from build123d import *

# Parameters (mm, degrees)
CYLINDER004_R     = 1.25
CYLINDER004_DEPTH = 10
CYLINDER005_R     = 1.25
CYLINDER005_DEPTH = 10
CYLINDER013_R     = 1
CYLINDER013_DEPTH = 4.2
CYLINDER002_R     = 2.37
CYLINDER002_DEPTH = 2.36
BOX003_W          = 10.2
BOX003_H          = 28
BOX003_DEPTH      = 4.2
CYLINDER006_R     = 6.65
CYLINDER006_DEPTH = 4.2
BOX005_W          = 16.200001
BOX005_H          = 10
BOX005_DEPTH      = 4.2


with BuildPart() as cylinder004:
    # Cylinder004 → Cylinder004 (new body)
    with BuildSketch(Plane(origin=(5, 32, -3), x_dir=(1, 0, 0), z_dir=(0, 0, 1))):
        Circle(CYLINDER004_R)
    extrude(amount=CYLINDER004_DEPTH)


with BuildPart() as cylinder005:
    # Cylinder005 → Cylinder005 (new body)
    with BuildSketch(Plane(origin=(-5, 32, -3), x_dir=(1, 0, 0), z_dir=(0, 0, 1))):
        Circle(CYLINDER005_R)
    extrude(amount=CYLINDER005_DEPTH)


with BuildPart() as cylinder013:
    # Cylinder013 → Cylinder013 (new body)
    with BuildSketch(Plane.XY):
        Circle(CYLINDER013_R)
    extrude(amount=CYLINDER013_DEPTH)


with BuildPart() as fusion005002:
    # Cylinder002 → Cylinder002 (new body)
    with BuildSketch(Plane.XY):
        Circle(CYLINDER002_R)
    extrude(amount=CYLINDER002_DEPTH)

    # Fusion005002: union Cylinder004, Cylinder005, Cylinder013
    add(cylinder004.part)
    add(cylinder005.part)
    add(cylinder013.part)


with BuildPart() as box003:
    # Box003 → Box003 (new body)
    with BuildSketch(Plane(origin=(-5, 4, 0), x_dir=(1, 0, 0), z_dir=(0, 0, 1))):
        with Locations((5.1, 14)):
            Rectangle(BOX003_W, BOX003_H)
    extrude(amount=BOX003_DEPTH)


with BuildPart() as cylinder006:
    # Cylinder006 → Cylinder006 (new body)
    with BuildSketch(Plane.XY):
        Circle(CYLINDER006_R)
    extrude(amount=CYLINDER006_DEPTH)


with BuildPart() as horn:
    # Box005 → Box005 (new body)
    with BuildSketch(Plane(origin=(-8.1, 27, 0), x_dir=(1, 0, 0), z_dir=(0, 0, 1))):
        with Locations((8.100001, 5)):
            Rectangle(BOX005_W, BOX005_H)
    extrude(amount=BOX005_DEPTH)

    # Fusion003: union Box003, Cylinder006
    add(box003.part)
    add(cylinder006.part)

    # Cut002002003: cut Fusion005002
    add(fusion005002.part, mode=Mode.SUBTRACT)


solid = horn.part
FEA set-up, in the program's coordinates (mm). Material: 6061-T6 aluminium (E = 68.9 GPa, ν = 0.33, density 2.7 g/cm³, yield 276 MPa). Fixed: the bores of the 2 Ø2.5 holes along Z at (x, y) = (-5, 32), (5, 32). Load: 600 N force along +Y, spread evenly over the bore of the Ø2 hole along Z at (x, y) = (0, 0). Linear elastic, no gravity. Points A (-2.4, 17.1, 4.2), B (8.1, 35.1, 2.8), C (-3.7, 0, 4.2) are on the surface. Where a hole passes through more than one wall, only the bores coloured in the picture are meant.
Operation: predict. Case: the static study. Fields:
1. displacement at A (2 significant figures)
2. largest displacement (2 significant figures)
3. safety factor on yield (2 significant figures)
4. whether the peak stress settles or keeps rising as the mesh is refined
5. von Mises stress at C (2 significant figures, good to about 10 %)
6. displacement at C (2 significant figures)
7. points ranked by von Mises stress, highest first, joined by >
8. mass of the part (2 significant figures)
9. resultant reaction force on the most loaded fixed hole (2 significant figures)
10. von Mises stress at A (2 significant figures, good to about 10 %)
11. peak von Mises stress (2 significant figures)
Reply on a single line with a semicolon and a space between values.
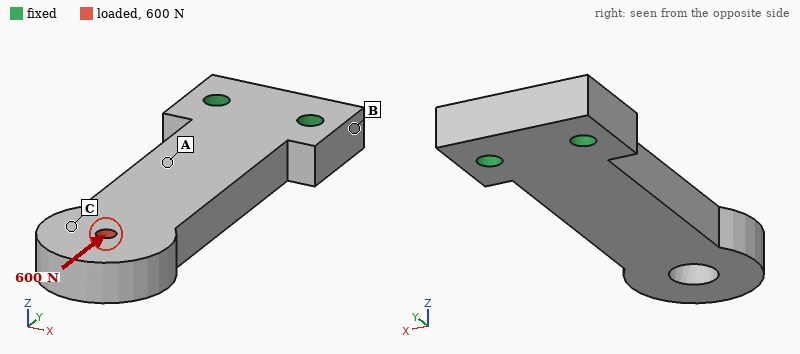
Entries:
0.018 mm; 0.11 mm; 2.7; settles; 16 MPa; 0.079 mm; A > C > B; 5.6 g; 310 N; 38 MPa; 100 MPa
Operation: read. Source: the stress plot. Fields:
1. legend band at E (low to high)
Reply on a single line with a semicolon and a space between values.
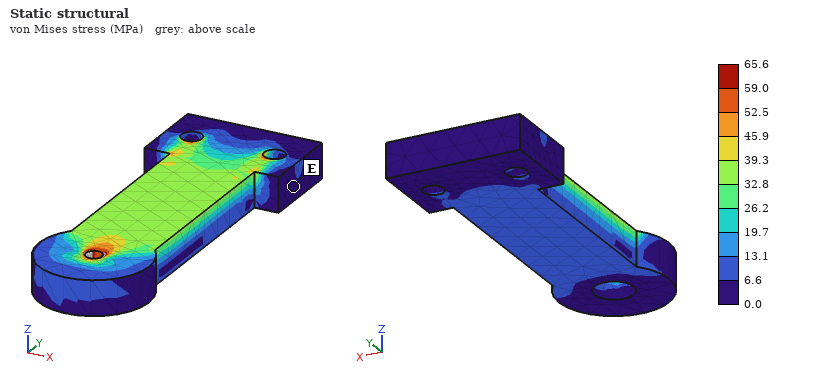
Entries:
0.0 to 6.6 MPa
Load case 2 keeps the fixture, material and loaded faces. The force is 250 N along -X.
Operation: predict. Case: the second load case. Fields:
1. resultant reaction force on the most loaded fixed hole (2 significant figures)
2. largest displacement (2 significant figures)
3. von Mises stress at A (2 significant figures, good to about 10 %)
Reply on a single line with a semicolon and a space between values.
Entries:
760 N; 0.12 mm; 36 MPa
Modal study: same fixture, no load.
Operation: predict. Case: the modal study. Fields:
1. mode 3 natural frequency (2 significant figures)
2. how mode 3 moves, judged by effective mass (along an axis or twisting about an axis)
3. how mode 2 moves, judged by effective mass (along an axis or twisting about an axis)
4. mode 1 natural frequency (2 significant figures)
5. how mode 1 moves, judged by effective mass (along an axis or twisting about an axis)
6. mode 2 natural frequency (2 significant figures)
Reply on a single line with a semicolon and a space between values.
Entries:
13 kHz; twisting about Y; along X; 2400 Hz; along Z; 6100 Hz
